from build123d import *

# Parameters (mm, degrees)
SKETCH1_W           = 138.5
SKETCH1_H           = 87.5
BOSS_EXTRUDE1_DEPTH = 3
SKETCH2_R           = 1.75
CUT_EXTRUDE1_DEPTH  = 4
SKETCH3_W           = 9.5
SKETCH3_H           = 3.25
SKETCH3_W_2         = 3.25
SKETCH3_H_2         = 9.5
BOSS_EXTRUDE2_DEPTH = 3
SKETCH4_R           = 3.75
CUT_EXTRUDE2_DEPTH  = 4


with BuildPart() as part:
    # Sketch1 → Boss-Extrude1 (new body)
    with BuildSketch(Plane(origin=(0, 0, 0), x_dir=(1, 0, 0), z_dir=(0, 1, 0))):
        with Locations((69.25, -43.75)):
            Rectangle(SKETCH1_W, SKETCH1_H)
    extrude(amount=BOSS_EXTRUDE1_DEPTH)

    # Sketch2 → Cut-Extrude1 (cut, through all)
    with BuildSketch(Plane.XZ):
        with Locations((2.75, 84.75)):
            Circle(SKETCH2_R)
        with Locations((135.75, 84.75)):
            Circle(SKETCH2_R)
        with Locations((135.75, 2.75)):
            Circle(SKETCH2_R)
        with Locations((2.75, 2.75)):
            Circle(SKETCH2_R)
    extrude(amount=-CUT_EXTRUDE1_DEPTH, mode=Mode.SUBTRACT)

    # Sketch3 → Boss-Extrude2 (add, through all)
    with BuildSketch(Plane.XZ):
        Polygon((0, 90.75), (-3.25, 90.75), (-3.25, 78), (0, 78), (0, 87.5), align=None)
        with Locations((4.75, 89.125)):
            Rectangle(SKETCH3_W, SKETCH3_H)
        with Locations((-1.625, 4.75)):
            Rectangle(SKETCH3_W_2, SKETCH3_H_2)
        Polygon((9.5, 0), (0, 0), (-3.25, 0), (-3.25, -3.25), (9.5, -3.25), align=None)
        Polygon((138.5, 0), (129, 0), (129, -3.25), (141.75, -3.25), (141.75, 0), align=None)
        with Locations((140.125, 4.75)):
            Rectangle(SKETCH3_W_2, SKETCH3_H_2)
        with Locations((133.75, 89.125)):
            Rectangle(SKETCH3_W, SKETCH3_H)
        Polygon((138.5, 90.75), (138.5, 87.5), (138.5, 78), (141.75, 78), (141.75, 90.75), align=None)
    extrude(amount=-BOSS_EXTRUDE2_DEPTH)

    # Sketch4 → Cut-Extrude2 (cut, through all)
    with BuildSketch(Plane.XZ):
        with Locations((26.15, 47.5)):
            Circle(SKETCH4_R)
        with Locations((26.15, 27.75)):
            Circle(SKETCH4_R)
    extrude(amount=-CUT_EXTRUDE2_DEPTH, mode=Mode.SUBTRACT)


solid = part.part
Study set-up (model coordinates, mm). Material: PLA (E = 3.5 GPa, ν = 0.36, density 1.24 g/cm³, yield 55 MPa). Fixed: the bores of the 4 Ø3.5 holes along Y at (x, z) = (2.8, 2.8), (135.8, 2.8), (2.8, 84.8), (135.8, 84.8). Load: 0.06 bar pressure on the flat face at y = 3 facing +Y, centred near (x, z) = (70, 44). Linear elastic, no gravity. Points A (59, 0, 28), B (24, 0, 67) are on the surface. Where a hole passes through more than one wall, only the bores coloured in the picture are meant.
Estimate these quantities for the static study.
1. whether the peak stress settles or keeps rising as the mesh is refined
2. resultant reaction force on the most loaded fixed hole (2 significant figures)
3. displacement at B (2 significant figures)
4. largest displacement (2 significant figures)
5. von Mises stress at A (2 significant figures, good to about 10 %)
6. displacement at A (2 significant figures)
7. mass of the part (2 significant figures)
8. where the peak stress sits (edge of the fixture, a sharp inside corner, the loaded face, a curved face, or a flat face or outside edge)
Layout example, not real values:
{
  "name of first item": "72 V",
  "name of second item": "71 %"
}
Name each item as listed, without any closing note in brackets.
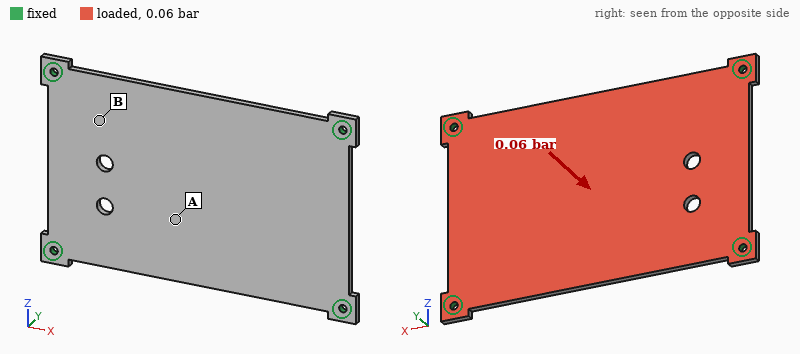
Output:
{
  "whether the peak stress settles or keeps rising as the mesh is refined": "keeps rising",
  "resultant reaction force on the most loaded fixed hole": "19 N",
  "displacement at B": "0.45 mm",
  "largest displacement": "1.0 mm",
  "von Mises stress at A": "3.3 MPa",
  "displacement at A": "1.0 mm",
  "mass of the part": "46 g",
  "where the peak stress sits": "edge of the fixture"
}
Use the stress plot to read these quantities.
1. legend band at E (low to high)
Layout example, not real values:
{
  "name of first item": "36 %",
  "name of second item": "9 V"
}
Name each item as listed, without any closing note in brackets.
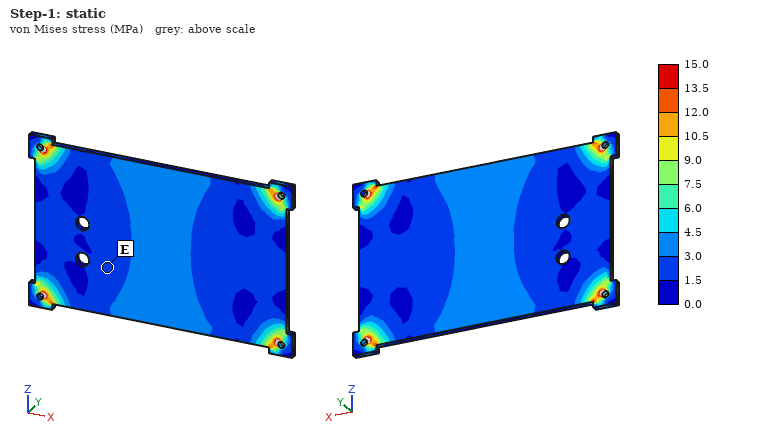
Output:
{
  "legend band at E": "1.5 to 3.0 MPa"
}
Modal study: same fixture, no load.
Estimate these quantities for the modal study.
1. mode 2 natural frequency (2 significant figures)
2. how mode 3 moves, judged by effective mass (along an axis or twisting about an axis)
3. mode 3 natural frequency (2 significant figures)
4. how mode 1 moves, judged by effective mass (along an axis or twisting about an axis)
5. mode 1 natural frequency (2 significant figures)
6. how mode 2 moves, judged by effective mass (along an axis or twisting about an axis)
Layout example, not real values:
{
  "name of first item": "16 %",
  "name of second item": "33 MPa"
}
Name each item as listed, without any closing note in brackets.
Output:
{
  "mode 2 natural frequency": "400 Hz",
  "how mode 3 moves, judged by effective mass": "twisting about Z",
  "mode 3 natural frequency": "590 Hz",
  "how mode 1 moves, judged by effective mass": "along Y",
  "mode 1 natural frequency": "230 Hz",
  "how mode 2 moves, judged by effective mass": "twisting about X"
}
